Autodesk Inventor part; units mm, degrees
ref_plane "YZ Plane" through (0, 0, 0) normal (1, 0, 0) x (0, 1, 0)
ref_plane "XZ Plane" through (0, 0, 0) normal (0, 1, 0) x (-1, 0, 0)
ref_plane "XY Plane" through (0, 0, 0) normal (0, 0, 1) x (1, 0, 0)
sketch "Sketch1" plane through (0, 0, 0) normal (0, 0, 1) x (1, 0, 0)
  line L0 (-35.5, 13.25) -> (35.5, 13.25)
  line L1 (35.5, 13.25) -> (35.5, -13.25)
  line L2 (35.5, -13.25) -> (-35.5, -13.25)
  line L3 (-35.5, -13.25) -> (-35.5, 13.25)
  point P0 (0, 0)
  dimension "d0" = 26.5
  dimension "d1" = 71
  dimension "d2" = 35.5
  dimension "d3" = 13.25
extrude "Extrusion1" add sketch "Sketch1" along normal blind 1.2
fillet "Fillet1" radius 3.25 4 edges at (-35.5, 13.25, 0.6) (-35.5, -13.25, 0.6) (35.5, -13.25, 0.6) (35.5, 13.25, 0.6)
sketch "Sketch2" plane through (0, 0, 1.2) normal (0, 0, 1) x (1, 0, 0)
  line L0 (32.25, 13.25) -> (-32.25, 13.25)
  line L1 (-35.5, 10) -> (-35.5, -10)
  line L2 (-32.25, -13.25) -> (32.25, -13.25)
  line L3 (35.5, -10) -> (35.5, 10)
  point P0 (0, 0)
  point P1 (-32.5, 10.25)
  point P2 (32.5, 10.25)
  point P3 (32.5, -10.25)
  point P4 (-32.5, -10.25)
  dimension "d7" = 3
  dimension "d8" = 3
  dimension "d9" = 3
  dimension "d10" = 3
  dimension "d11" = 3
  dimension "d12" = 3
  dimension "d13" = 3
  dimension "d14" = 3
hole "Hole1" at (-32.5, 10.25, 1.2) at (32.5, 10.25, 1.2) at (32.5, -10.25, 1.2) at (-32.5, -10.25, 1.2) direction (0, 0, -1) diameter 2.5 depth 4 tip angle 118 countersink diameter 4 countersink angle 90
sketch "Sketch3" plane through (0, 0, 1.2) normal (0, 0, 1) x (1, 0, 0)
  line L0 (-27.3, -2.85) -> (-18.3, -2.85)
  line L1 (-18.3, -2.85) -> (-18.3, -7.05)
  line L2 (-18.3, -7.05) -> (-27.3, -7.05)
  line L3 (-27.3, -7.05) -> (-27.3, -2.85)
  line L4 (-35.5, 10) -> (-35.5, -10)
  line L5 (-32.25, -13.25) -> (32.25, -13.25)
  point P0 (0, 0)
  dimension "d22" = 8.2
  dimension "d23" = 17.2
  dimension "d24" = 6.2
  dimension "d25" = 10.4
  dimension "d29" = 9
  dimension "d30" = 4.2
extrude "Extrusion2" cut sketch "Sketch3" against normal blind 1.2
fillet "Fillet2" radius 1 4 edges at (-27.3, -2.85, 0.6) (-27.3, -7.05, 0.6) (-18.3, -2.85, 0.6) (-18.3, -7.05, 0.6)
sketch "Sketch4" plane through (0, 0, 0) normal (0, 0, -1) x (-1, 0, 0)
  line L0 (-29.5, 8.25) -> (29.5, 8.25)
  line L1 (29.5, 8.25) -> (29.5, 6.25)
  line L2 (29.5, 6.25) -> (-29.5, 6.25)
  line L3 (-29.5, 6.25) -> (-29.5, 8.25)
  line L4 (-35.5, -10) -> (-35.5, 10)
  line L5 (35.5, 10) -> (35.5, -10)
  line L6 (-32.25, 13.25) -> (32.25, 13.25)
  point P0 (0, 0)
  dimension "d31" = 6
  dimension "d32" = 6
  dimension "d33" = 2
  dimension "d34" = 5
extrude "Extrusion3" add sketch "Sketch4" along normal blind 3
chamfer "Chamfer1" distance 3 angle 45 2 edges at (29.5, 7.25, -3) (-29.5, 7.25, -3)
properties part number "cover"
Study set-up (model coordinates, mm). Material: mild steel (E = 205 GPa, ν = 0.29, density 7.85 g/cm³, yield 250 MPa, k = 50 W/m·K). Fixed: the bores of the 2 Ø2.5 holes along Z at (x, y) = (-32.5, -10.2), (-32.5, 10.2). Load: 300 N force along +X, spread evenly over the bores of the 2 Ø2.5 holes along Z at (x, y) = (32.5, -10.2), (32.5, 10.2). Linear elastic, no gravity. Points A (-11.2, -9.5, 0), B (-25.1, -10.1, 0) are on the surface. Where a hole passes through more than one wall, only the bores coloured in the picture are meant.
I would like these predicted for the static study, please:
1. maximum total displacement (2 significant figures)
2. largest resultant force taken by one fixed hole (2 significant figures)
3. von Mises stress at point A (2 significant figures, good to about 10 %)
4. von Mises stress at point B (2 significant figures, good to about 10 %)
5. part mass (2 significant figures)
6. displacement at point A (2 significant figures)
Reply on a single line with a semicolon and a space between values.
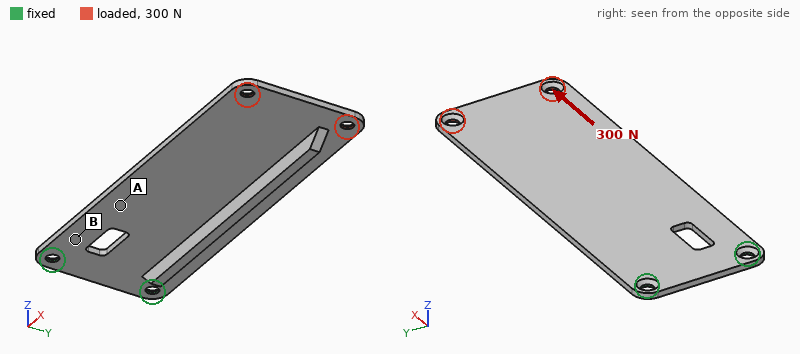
84 µm; 150 N; 12 MPa; 26 MPa; 20 g; 14 µm
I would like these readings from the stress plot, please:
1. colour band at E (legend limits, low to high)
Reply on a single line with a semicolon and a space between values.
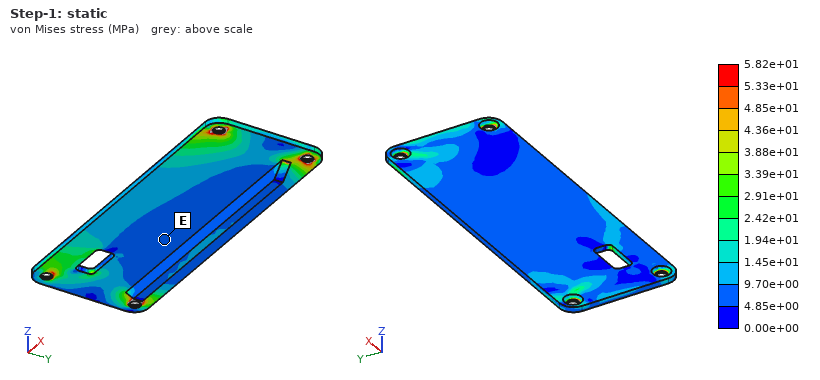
4.85e+00 to 9.70e+00 MPa
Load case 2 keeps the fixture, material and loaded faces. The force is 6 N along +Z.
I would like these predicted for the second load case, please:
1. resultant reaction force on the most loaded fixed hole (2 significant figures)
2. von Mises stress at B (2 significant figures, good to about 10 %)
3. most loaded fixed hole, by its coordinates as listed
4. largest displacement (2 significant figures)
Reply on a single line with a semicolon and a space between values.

5.2 N; 39 MPa; (-32.5, -10.2); 0.40 mm
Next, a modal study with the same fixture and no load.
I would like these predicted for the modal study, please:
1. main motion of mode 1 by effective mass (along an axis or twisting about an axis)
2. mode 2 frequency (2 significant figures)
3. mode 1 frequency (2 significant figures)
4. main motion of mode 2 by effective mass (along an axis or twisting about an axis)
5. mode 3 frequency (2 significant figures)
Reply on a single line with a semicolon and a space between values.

along Z; 1300 Hz; 260 Hz; twisting about X; 2300 Hz
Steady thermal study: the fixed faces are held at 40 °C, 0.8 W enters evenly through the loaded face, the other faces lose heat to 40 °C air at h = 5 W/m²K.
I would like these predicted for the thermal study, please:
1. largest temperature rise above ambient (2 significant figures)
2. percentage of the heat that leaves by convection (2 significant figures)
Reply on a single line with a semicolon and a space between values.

28 K; 32 %
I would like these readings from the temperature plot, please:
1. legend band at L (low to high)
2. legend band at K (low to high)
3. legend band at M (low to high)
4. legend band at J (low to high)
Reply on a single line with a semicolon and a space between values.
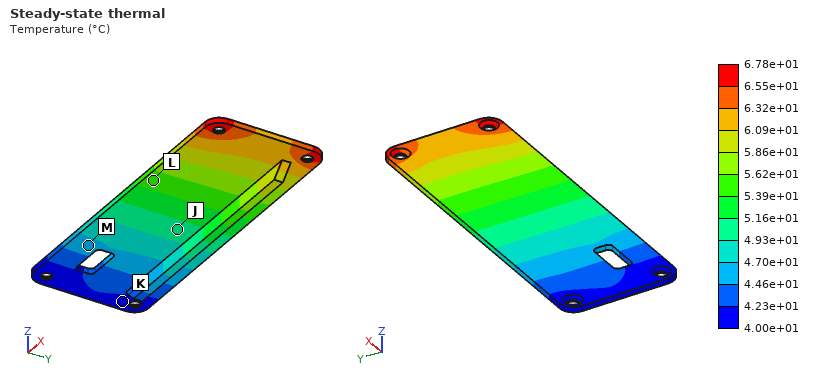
5.39e+01 to 5.62e+01 °C; 4.00e+01 to 4.23e+01 °C; 4.46e+01 to 4.70e+01 °C; 4.93e+01 to 5.16e+01 °C
